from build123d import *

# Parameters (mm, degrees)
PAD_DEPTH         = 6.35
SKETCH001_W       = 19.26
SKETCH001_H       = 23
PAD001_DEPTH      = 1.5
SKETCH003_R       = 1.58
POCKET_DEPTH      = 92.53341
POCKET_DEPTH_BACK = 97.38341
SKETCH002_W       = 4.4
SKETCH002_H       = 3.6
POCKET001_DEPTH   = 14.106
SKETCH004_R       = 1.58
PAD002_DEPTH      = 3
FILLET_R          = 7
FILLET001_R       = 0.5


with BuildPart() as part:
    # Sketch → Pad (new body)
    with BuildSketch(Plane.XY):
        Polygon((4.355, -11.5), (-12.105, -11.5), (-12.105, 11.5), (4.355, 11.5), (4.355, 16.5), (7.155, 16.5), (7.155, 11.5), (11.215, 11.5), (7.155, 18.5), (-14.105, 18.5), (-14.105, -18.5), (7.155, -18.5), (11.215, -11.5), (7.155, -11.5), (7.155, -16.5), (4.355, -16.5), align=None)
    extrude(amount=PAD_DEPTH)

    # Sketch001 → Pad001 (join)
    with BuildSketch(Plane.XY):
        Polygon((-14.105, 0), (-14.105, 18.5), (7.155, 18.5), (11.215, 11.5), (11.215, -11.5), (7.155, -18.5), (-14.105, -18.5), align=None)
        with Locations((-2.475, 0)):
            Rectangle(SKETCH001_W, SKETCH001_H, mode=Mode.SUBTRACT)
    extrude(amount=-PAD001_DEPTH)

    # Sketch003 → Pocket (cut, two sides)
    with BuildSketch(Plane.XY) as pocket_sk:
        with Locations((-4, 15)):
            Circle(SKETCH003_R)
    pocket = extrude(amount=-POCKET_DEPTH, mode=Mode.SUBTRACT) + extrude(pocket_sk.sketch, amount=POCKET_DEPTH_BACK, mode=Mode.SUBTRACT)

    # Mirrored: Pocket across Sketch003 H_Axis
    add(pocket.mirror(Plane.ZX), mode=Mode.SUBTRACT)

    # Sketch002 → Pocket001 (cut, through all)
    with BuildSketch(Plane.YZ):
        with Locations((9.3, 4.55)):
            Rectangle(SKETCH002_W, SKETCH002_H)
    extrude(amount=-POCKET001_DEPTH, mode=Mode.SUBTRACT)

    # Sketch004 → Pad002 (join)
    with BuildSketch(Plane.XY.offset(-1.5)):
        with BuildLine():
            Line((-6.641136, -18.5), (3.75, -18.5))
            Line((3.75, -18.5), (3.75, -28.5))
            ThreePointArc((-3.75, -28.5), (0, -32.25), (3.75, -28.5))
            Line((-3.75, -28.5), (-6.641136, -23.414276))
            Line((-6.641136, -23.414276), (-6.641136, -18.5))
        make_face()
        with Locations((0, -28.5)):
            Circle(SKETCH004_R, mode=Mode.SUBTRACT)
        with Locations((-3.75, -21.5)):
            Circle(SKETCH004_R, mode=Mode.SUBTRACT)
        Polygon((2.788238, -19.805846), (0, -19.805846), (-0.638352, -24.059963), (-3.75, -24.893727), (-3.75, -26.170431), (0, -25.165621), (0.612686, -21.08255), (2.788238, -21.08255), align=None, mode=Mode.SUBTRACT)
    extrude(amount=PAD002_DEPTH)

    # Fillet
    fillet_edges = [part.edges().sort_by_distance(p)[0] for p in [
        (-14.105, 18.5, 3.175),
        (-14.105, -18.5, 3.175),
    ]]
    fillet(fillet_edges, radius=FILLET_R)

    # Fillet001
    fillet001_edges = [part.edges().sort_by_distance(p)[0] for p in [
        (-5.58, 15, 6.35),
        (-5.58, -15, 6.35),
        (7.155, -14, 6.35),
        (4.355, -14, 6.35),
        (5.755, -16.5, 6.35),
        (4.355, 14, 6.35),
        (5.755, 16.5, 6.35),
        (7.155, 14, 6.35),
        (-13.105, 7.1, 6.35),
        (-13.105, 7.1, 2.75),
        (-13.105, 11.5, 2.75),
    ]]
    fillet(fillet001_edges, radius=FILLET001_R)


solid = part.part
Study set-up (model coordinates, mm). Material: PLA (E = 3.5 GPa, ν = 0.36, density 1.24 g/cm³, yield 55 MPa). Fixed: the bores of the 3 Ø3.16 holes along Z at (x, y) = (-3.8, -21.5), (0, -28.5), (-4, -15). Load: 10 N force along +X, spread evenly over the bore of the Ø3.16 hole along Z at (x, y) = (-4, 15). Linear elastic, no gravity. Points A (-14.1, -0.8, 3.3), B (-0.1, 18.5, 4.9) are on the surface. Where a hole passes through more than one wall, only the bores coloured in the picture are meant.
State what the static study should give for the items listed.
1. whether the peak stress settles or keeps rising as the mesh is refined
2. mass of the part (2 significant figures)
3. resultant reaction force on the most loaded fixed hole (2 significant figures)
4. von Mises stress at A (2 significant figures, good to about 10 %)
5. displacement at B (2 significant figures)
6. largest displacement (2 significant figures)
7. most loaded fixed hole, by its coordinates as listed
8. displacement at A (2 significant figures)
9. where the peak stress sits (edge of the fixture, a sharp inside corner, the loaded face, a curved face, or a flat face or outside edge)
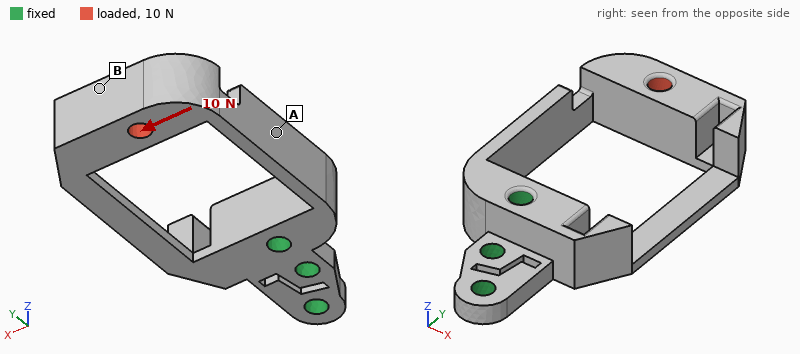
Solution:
keeps rising
3.5 g
29 N
2.8 MPa
0.55 mm
0.57 mm
(-4, -15)
0.21 mm
a sharp inside corner
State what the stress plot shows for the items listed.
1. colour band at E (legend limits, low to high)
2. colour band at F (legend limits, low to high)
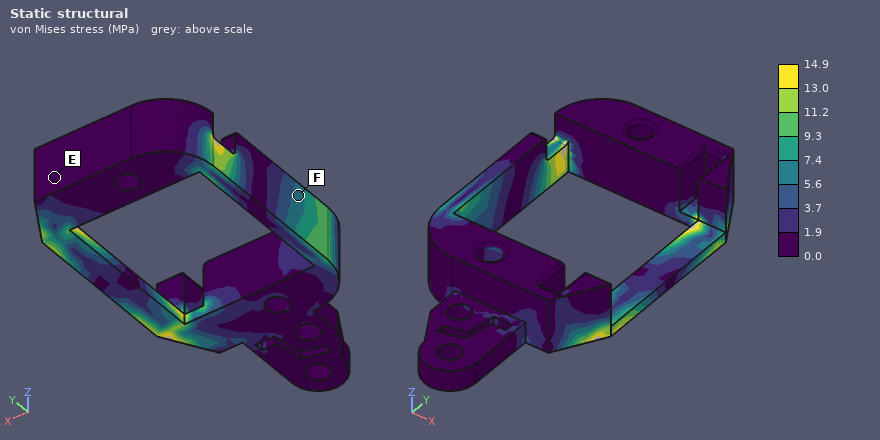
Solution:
0.0 to 1.9 MPa
5.6 to 7.4 MPa
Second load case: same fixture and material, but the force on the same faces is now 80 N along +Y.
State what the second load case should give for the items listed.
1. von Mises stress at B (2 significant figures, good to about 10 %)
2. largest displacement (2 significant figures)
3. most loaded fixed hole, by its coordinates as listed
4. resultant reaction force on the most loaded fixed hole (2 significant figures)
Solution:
4.3 MPa
0.66 mm
(-4, -15)
41 N
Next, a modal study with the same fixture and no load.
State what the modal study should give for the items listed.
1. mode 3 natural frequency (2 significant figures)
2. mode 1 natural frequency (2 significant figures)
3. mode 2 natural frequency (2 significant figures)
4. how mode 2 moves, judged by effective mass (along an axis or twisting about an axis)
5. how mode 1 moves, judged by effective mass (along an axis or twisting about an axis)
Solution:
1200 Hz
400 Hz
590 Hz
along X
along Z
